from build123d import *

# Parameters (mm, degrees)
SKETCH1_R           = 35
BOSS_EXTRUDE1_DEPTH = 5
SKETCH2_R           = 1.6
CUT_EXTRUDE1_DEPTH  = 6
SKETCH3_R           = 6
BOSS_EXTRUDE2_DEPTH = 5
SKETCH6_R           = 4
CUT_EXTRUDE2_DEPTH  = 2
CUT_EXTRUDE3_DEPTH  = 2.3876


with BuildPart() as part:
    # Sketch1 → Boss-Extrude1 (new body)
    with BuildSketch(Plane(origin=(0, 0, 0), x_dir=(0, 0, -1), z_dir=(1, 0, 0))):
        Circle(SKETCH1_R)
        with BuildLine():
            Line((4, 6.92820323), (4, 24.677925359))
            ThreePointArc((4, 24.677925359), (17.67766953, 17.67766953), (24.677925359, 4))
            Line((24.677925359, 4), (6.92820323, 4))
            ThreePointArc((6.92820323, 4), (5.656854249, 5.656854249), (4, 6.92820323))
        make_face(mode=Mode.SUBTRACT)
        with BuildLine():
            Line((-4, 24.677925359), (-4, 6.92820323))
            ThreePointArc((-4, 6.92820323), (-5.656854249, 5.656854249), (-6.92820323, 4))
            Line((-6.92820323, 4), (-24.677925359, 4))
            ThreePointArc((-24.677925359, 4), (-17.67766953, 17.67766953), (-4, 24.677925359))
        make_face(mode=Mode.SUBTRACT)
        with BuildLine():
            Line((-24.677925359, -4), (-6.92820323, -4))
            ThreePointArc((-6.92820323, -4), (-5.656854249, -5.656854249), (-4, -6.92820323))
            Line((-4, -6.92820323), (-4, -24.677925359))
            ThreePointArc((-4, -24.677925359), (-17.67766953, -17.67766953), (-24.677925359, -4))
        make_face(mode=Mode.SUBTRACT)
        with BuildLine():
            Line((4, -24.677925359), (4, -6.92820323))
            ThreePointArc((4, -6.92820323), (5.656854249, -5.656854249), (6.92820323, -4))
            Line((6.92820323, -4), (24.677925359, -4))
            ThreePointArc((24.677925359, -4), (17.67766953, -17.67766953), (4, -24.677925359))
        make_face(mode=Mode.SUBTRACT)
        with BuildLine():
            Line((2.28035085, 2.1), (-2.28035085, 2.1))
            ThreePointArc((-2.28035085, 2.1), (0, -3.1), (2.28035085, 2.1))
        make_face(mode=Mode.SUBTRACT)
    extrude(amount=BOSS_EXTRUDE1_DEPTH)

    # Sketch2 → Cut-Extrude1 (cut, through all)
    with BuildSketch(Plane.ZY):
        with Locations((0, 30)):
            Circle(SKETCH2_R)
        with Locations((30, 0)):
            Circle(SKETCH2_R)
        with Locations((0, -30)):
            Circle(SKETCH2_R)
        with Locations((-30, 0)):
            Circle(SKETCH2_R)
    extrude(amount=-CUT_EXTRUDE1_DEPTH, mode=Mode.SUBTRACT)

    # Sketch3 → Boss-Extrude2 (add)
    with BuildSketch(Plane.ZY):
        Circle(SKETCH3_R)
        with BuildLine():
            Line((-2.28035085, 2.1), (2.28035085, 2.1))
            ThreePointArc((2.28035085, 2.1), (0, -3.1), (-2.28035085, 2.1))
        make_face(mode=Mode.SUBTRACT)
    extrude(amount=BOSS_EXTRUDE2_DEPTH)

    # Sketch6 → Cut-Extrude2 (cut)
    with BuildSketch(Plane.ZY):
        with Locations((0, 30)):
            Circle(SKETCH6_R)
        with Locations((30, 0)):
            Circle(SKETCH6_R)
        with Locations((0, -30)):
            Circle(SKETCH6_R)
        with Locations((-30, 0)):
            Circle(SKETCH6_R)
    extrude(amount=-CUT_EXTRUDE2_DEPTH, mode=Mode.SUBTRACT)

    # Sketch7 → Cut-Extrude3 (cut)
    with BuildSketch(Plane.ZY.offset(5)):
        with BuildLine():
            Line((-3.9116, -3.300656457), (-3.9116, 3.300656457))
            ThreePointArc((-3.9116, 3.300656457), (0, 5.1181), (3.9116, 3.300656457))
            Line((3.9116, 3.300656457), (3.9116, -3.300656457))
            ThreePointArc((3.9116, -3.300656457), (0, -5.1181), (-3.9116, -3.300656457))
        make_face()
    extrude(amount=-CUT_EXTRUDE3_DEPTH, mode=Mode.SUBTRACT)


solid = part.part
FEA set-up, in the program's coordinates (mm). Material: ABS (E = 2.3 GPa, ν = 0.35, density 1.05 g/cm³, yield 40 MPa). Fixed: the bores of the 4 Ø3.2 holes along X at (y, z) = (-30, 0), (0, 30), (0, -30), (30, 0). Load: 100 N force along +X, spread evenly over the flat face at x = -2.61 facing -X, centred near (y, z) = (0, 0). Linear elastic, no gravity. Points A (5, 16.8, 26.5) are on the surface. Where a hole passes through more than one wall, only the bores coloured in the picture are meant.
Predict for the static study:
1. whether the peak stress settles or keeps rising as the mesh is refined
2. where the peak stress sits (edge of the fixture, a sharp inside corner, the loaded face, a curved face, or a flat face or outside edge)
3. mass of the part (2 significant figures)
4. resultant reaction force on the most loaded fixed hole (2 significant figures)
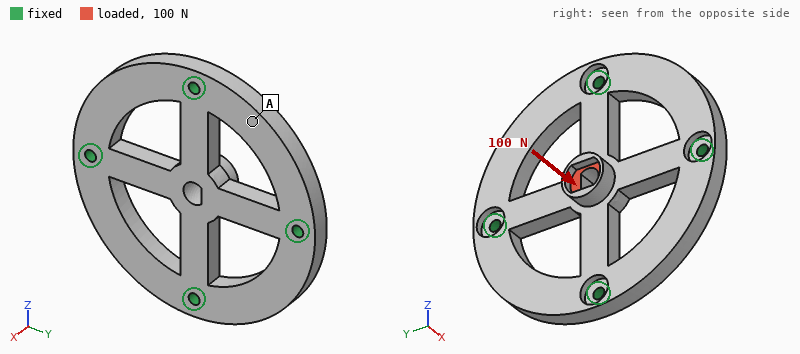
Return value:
keeps rising
edge of the fixture
14 g
44 N
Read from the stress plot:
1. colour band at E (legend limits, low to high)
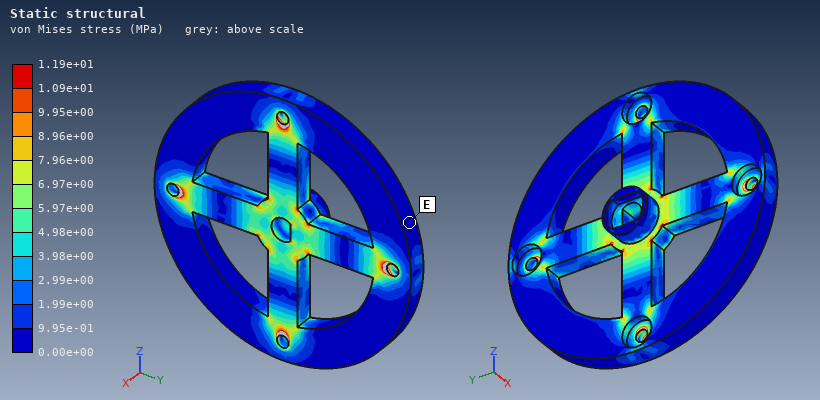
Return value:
0.00e+00 to 9.95e-01 MPa
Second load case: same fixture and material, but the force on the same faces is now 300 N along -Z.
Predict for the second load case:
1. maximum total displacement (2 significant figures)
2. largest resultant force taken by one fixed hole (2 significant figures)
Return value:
0.18 mm
140 N
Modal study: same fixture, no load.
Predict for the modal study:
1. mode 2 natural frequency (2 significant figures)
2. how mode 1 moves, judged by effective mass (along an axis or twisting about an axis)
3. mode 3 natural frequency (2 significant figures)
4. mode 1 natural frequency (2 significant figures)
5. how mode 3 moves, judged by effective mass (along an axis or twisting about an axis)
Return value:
2200 Hz
along X
2400 Hz
2100 Hz
twisting about Y
